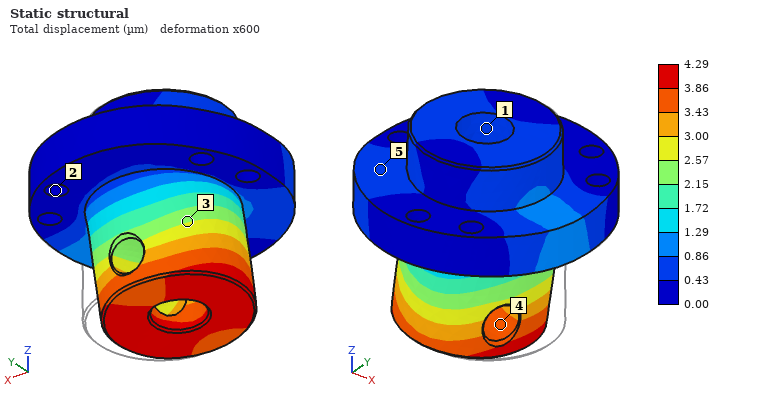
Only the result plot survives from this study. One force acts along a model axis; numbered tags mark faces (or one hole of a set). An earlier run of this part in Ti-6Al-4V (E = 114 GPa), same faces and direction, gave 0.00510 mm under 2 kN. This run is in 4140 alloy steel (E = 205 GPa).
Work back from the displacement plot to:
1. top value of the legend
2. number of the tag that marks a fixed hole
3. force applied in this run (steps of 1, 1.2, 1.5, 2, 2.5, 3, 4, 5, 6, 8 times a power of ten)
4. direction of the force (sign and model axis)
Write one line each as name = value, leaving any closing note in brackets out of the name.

top value of the legend = 4.29 µm
number of the tag that marks a fixed hole = 2
force applied in this run = 3 kN
direction of the force = -X
